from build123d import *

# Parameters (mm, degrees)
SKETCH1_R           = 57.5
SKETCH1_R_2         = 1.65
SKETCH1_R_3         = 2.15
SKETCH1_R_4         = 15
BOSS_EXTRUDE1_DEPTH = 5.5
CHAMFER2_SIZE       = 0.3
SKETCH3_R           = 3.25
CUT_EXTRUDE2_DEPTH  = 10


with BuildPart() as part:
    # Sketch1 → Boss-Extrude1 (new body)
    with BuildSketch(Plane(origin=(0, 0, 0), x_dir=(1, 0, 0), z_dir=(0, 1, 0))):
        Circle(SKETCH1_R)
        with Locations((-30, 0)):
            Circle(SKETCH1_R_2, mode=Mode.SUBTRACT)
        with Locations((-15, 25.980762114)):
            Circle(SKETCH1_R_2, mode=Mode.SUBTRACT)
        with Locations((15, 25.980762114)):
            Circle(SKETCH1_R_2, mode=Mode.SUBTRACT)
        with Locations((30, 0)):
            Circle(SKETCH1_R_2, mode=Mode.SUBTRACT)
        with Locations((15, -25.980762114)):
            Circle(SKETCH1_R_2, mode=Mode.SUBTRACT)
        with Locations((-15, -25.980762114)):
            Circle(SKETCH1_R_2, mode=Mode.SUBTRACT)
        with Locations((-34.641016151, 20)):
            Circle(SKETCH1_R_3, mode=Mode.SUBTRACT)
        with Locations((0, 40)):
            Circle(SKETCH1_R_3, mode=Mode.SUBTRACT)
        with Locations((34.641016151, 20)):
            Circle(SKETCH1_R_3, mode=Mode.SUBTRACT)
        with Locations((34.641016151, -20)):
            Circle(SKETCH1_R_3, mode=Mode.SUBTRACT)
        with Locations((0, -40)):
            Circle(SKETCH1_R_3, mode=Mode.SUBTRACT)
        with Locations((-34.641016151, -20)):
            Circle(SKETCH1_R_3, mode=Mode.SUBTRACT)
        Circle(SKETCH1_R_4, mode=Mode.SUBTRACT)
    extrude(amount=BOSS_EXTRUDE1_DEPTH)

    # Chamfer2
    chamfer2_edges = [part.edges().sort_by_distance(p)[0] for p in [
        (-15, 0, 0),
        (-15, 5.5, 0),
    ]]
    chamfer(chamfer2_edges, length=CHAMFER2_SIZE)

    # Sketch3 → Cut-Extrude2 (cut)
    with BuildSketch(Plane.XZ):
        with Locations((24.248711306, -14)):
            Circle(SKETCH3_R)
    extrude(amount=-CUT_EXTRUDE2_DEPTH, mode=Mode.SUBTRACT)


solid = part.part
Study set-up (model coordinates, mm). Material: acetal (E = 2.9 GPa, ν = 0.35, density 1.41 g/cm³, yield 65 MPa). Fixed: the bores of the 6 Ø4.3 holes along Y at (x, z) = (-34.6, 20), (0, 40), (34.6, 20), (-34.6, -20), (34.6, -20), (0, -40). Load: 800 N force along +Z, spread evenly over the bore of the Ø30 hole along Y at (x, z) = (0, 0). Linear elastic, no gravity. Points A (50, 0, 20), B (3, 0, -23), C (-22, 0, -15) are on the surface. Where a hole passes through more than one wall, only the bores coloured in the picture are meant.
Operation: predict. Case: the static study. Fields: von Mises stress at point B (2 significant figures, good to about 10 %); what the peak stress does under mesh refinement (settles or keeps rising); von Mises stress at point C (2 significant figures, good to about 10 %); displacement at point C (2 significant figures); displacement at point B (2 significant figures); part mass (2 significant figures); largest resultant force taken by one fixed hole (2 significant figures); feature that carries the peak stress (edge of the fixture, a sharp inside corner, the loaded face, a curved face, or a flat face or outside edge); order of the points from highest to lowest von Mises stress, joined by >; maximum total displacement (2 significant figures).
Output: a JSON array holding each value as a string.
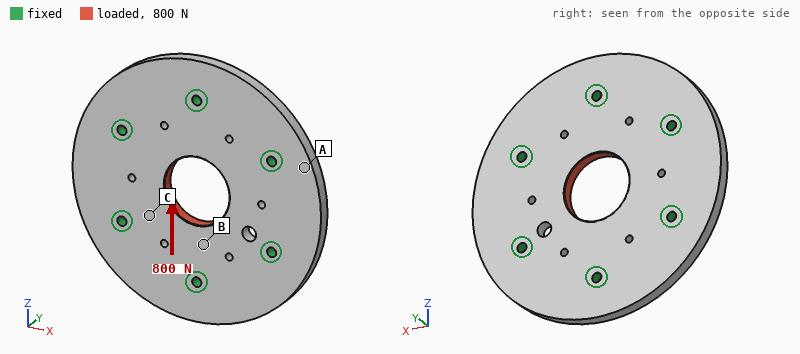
["1.6 MPa", "keeps rising", "0.98 MPa", "8.1 µm", "12 µm", "74 g", "200 N", "edge of the fixture", "B > C > A", "18 µm"]
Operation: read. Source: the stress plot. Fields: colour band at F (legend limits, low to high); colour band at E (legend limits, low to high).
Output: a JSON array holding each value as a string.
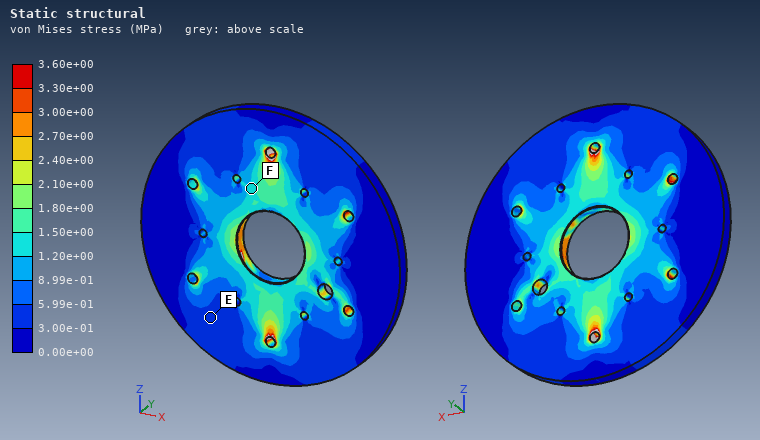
["1.20e+00 to 1.50e+00 MPa", "3.00e-01 to 5.99e-01 MPa"]
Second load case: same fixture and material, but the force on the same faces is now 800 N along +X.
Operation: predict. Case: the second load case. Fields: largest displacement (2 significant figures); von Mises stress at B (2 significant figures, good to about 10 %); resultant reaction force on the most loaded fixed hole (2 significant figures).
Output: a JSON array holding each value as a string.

["19 µm", "0.89 MPa", "170 N"]
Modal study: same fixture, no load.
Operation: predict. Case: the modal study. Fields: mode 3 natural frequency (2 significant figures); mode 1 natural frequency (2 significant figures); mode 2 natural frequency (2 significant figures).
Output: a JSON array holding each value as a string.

["2300 Hz", "2100 Hz", "2200 Hz"]
